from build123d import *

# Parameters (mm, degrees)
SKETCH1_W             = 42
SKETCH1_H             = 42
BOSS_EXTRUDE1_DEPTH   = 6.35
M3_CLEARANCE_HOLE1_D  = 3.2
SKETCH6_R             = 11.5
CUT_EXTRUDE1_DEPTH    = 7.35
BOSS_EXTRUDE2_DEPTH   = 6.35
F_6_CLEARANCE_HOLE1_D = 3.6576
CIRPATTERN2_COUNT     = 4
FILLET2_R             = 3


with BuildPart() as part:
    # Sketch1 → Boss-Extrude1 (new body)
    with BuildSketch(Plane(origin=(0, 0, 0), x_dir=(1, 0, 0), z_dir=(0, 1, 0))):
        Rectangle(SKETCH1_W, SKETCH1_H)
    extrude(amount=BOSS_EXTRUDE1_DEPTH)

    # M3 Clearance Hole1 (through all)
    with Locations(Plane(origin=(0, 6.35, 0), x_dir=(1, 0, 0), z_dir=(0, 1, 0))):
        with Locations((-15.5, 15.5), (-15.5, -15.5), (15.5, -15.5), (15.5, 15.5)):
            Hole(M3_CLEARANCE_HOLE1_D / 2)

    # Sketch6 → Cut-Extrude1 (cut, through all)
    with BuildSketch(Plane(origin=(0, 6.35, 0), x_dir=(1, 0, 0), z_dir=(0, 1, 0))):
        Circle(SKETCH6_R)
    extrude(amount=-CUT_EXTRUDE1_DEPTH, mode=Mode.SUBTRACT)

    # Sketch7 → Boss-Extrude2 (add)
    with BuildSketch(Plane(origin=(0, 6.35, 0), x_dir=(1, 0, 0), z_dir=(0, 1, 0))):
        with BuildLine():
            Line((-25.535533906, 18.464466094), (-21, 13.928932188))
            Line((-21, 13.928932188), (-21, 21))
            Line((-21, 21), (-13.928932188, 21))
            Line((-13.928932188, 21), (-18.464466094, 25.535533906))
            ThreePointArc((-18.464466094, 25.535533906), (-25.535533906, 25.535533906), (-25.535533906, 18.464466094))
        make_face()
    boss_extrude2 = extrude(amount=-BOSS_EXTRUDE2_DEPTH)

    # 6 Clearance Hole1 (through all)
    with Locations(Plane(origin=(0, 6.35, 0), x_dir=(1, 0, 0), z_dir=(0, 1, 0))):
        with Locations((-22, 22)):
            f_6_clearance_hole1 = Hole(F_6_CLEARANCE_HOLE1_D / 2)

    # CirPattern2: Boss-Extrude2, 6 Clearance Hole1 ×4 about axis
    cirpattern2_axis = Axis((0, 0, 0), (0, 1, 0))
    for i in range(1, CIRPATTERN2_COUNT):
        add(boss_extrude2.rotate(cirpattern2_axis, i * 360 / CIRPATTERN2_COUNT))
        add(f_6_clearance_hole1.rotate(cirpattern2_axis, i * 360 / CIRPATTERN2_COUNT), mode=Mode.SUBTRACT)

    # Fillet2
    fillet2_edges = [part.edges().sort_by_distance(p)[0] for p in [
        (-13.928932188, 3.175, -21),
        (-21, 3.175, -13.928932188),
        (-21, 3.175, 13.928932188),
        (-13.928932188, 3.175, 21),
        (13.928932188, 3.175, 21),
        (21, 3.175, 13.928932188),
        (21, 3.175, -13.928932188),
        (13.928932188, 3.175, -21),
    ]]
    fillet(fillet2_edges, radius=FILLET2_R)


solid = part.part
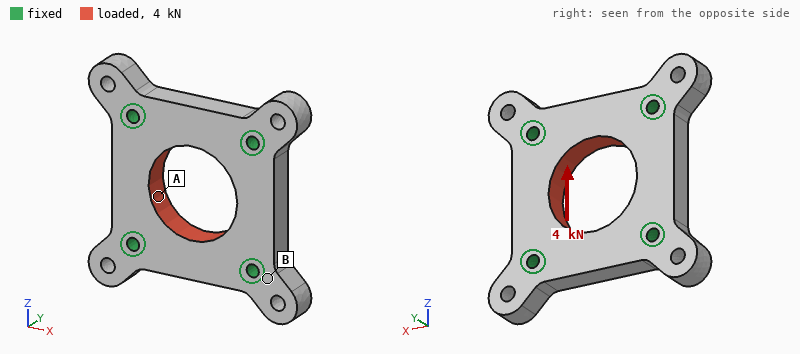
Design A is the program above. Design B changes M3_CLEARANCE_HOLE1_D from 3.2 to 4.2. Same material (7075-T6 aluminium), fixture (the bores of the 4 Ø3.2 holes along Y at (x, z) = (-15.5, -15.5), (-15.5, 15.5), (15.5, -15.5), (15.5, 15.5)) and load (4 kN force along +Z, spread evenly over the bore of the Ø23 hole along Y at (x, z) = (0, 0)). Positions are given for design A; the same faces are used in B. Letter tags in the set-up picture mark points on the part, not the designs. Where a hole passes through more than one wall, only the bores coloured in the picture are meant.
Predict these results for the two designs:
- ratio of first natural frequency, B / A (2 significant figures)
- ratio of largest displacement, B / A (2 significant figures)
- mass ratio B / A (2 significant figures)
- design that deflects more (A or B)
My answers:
1.1
0.92
0.99
A
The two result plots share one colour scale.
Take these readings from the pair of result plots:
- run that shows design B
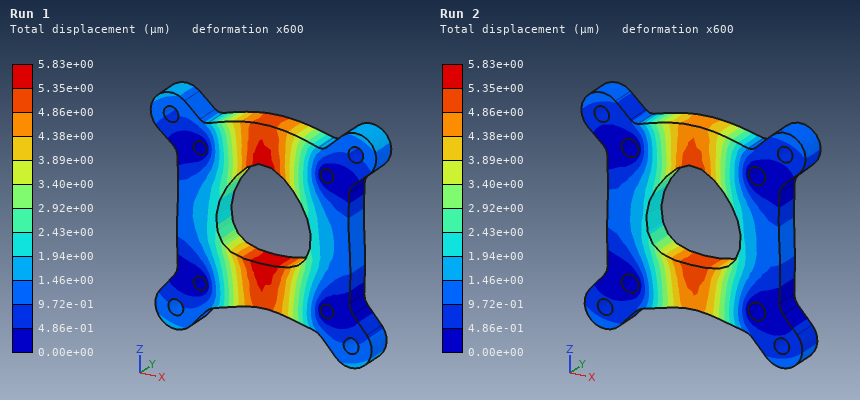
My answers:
Run 2
